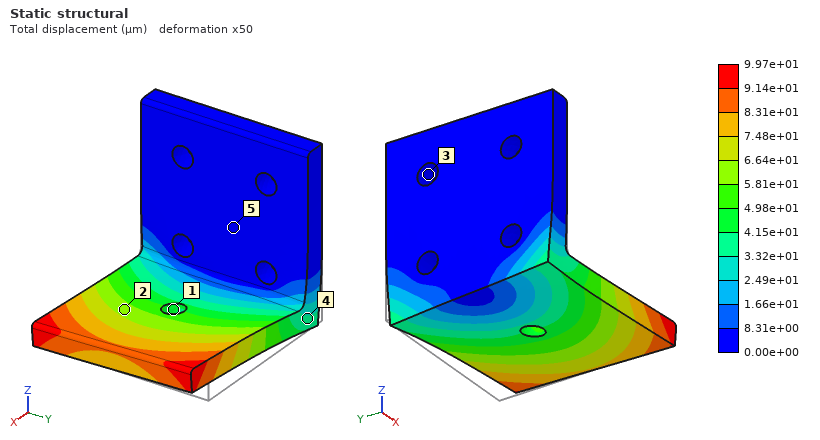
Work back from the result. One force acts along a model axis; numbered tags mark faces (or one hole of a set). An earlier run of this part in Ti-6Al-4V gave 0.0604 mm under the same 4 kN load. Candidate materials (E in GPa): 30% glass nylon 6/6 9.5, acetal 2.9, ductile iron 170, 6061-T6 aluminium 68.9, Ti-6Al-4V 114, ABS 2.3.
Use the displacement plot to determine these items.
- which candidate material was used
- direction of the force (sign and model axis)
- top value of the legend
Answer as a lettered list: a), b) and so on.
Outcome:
a) 6061-T6 aluminium
b) -Y
c) 9.97e+01 µm
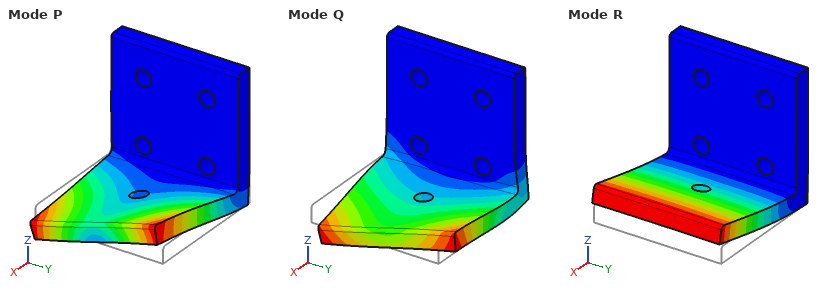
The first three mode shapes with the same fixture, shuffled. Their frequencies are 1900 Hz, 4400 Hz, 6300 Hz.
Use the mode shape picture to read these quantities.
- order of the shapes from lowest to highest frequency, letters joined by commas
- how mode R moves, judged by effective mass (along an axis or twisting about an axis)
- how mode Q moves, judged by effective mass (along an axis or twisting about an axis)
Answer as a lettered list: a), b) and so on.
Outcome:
a) R, P, Q
b) along Z
c) along Y
